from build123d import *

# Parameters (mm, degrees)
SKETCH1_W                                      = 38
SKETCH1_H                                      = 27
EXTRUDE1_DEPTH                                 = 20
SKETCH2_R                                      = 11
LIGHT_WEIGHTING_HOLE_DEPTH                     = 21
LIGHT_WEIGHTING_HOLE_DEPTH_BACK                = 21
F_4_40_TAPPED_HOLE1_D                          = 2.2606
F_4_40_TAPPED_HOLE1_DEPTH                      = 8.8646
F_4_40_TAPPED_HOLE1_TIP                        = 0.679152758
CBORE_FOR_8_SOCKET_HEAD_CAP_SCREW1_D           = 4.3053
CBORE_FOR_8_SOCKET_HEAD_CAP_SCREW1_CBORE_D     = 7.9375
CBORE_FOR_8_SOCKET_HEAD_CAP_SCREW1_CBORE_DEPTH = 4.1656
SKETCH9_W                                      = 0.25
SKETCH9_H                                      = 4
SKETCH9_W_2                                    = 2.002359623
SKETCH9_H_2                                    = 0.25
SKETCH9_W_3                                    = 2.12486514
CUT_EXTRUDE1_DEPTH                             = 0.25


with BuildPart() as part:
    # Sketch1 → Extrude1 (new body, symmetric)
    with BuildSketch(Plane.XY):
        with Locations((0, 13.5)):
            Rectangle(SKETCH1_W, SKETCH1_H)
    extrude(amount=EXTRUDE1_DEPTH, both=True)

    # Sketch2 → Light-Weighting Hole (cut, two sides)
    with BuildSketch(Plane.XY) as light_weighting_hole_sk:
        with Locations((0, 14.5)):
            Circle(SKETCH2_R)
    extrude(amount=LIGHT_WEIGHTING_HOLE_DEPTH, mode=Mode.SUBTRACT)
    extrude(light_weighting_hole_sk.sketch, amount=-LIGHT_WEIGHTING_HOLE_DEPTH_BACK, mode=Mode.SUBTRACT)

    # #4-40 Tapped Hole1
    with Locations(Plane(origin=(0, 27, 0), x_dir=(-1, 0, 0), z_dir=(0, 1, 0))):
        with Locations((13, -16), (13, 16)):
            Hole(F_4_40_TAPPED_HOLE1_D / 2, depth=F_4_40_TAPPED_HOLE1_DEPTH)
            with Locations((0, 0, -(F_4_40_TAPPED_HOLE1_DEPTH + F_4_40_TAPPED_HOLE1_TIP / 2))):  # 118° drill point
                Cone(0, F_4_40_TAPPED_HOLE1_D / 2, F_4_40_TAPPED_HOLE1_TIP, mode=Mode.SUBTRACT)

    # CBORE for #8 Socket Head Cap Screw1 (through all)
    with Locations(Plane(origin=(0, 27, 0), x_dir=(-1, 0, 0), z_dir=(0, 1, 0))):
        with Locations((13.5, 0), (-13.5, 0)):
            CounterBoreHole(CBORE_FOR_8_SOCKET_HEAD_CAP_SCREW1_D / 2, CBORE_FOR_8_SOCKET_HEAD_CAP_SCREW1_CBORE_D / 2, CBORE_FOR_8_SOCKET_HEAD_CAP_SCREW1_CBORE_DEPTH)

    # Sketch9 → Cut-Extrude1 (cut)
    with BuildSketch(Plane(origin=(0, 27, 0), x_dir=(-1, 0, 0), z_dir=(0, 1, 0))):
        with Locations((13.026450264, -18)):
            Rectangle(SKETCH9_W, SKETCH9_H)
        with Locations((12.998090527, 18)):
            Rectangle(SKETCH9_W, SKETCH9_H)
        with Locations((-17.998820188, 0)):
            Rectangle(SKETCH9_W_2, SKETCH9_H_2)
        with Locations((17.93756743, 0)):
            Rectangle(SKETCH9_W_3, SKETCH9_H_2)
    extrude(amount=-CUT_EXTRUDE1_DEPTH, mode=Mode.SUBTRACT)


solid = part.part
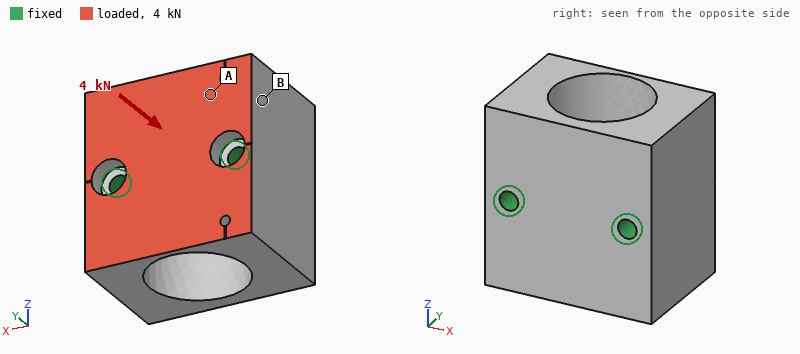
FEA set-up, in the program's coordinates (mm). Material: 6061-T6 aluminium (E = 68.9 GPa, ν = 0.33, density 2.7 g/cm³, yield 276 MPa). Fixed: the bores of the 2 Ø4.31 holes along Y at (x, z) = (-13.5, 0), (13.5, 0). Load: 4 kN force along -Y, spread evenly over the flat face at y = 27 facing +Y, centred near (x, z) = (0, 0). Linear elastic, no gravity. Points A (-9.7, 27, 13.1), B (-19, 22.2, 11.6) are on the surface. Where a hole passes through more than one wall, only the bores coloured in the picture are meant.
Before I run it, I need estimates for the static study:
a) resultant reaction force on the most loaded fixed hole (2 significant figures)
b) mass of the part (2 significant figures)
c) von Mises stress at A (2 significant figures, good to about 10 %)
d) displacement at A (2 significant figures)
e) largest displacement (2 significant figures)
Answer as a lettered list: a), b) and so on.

a) 2.1 kN
b) 67 g
c) 11 MPa
d) 4.5 µm
e) 13 µm
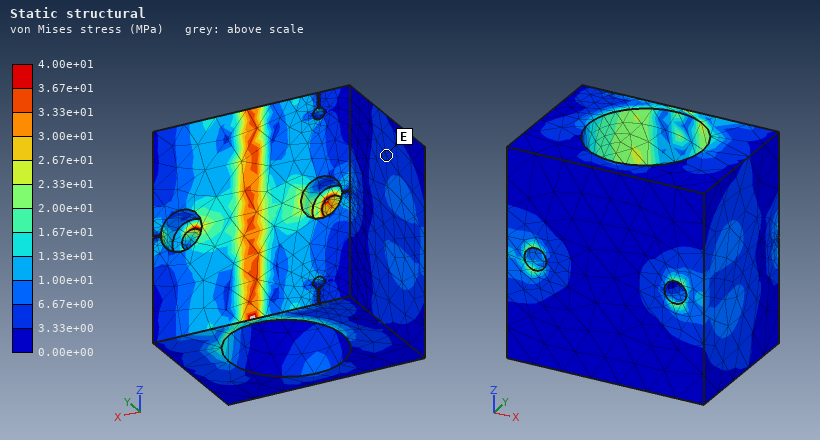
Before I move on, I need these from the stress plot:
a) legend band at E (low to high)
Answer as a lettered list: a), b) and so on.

a) 3.33e+00 to 6.67e+00 MPa
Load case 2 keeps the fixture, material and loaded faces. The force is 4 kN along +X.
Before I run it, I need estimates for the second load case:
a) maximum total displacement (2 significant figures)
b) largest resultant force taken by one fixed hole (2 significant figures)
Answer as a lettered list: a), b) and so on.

a) 13 µm
b) 2.1 kN
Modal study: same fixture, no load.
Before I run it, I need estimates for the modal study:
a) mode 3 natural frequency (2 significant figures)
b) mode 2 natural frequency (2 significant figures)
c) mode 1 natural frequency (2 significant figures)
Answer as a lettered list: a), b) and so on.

a) 24 kHz
b) 23 kHz
c) 22 kHz
